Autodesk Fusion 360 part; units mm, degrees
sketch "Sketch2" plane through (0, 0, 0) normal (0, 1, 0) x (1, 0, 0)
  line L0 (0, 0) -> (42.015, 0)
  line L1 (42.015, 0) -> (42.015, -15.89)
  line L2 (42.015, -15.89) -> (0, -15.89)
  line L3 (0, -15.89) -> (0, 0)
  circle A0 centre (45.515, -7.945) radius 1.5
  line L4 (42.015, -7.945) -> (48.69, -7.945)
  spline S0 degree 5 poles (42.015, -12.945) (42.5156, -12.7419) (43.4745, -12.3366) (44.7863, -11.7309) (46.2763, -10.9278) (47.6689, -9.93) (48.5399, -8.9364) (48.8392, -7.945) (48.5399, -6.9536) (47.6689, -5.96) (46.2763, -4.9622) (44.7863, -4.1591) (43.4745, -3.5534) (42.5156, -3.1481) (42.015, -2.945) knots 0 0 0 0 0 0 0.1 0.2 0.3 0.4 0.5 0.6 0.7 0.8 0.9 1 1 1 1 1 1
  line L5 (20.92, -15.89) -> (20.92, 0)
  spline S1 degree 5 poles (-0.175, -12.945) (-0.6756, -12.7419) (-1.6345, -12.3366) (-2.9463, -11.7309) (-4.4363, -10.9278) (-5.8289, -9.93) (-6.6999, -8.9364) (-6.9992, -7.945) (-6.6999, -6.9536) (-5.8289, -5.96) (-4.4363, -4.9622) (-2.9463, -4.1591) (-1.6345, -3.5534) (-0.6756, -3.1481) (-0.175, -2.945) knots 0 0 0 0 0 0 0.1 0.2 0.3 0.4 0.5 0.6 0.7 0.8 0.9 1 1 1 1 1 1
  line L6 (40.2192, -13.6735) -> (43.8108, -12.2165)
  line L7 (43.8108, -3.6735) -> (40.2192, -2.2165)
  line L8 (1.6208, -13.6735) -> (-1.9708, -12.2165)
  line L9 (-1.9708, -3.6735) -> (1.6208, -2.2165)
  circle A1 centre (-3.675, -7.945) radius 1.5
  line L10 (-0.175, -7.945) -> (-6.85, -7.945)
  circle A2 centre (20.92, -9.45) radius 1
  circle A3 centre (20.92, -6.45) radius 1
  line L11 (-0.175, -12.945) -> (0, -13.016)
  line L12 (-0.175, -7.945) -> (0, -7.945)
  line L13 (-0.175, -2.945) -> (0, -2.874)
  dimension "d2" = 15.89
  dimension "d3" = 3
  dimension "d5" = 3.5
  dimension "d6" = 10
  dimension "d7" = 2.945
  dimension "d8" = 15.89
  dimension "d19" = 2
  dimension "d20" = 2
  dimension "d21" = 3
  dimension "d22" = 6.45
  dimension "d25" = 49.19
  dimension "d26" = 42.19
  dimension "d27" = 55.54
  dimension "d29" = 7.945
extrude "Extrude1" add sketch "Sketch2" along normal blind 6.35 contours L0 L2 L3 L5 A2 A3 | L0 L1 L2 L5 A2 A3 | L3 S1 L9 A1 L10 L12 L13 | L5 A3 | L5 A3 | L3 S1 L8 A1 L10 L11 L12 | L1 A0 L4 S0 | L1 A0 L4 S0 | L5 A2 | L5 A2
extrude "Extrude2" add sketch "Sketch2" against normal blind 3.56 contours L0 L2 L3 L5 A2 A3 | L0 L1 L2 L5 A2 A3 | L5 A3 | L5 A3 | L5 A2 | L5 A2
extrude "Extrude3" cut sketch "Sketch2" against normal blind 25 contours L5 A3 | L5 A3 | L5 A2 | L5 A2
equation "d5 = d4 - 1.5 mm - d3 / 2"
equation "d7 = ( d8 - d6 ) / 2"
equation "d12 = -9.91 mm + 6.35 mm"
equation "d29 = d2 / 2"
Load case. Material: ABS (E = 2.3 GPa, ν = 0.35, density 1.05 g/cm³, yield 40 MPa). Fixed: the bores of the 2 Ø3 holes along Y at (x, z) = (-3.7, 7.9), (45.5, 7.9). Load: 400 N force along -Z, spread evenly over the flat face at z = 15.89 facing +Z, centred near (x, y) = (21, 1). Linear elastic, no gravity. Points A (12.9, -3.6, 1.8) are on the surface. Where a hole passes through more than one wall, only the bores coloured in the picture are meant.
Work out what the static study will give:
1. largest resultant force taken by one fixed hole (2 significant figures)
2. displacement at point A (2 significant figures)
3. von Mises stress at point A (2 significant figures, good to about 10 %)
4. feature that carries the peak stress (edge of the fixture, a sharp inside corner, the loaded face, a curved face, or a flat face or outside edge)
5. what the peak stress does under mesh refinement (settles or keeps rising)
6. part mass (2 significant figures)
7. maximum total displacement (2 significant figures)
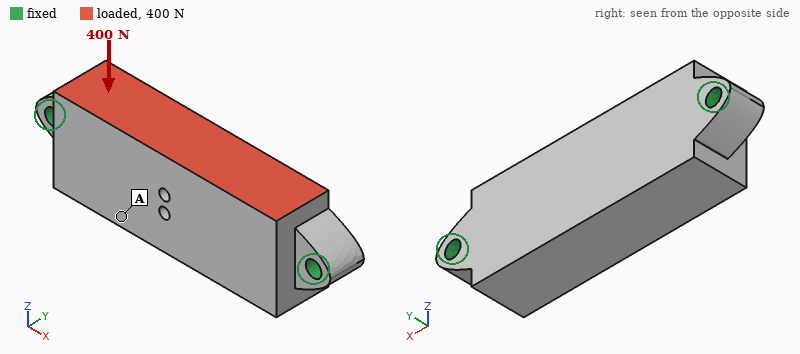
200 N
0.12 mm
3.4 MPa
edge of the fixture
keeps rising
7.4 g
0.13 mm
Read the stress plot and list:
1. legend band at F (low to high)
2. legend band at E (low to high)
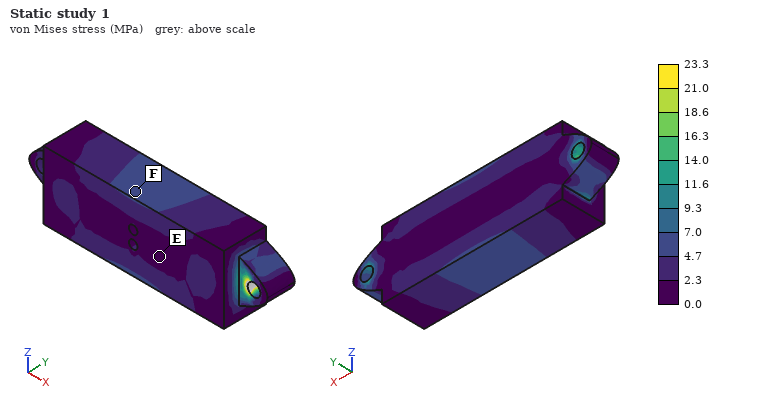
4.7 to 7.0 MPa
0.0 to 2.3 MPa
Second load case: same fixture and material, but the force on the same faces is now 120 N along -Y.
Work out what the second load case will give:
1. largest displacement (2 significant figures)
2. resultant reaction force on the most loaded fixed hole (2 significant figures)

0.11 mm
70 N
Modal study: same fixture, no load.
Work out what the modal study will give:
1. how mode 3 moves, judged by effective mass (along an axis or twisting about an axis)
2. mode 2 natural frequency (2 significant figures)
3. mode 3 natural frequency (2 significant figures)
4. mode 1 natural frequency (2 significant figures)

along Z
3700 Hz
4800 Hz
3600 Hz
